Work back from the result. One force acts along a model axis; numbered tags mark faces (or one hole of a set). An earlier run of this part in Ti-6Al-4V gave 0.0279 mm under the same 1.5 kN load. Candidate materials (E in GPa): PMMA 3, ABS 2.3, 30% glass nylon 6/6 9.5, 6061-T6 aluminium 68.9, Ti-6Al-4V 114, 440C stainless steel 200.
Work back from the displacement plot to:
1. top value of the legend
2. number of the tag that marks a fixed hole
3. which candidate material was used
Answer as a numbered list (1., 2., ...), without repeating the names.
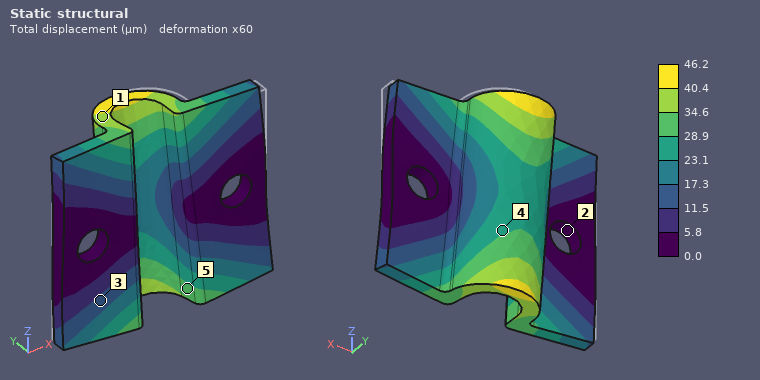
1. 46.2 µm
2. 2
3. 6061-T6 aluminium
